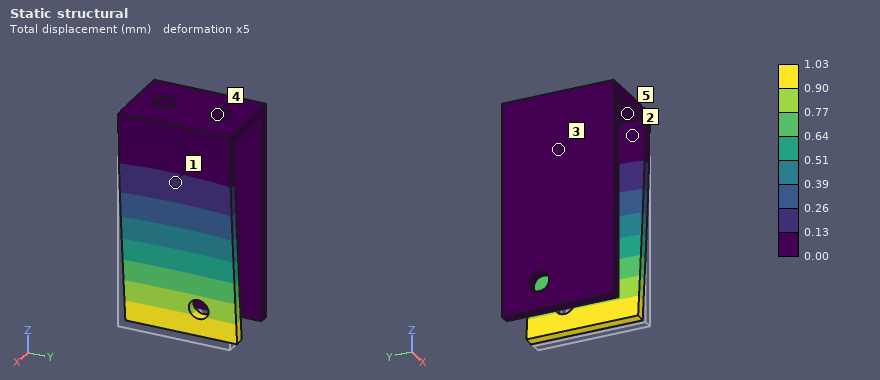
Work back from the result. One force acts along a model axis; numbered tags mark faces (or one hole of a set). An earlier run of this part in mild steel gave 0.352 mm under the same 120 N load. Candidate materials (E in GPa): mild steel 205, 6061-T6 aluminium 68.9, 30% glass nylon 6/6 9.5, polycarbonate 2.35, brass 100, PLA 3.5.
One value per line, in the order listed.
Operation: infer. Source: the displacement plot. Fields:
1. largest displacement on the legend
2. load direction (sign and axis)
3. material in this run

1.03 mm
-X
6061-T6 aluminium
